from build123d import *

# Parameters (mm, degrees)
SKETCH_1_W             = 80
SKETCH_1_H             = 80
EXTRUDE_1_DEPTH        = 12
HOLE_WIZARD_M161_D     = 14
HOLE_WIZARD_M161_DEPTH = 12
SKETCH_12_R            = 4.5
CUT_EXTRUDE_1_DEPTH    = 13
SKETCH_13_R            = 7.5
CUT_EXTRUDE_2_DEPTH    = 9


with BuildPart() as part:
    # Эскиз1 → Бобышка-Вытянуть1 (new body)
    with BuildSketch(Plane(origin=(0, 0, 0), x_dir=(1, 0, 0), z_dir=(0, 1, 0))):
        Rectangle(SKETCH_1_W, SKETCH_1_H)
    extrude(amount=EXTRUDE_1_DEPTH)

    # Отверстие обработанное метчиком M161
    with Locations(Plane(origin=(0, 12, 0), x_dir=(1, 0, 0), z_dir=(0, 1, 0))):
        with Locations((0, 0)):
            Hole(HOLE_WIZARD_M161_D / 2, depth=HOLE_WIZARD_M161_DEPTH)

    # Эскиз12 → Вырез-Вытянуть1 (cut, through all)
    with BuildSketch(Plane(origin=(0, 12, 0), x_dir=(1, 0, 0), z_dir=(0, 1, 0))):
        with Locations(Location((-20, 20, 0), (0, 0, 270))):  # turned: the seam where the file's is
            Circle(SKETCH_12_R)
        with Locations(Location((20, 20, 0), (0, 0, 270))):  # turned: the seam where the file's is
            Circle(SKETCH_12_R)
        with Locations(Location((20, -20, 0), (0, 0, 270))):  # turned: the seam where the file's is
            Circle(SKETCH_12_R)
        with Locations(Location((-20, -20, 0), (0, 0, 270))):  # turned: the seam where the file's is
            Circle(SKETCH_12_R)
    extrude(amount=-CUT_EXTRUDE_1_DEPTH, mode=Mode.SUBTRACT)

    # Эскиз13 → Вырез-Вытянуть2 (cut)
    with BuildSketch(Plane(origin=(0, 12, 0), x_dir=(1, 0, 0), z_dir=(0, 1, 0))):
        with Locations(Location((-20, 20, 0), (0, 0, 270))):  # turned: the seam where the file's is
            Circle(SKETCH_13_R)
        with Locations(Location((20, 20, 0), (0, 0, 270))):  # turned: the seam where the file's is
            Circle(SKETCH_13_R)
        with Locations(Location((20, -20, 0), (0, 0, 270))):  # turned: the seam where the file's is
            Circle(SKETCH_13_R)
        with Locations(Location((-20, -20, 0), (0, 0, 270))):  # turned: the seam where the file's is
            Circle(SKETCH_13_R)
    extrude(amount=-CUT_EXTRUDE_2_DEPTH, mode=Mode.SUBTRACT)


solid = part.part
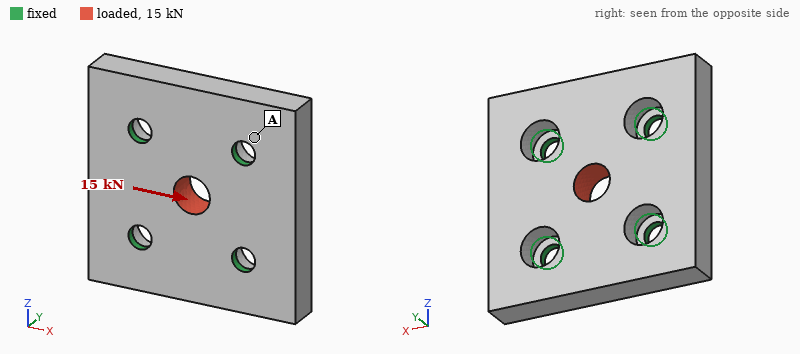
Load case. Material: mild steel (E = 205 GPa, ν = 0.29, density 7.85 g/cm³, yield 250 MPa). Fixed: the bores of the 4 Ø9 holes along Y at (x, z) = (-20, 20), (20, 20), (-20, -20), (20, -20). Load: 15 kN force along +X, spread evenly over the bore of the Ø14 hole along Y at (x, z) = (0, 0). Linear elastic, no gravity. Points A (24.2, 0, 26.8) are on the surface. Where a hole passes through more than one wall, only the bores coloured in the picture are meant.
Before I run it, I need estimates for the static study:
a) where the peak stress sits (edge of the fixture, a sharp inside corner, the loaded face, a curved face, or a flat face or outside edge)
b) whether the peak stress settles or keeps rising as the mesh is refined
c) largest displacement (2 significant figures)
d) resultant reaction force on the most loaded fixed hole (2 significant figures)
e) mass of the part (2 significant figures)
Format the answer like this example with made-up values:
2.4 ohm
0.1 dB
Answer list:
edge of the fixture
keeps rising
5.2 µm
3.9 kN
530 g
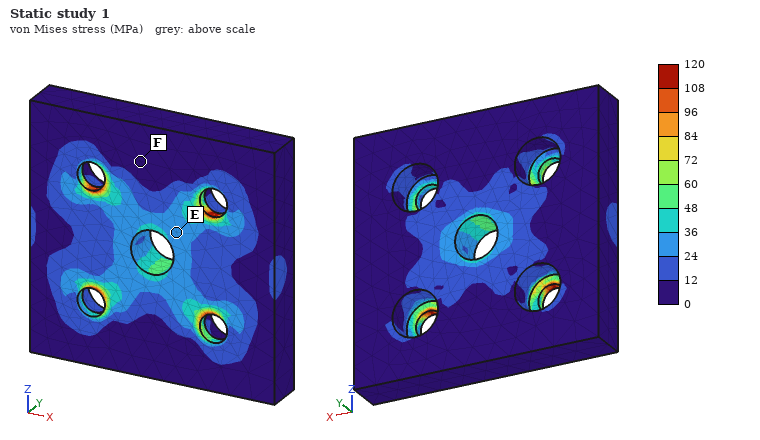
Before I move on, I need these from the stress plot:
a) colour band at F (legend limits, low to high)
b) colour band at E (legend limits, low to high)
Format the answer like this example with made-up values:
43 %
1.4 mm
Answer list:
0 to 12 MPa
24 to 36 MPa
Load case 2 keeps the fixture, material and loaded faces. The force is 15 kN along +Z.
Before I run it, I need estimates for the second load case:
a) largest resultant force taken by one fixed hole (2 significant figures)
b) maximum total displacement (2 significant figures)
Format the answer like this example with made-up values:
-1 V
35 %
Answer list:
3.9 kN
5.2 µm
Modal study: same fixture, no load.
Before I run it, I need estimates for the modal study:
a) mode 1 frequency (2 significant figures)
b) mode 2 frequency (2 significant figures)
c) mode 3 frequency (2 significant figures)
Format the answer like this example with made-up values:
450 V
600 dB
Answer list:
9900 Hz
9900 Hz
11 kHz
